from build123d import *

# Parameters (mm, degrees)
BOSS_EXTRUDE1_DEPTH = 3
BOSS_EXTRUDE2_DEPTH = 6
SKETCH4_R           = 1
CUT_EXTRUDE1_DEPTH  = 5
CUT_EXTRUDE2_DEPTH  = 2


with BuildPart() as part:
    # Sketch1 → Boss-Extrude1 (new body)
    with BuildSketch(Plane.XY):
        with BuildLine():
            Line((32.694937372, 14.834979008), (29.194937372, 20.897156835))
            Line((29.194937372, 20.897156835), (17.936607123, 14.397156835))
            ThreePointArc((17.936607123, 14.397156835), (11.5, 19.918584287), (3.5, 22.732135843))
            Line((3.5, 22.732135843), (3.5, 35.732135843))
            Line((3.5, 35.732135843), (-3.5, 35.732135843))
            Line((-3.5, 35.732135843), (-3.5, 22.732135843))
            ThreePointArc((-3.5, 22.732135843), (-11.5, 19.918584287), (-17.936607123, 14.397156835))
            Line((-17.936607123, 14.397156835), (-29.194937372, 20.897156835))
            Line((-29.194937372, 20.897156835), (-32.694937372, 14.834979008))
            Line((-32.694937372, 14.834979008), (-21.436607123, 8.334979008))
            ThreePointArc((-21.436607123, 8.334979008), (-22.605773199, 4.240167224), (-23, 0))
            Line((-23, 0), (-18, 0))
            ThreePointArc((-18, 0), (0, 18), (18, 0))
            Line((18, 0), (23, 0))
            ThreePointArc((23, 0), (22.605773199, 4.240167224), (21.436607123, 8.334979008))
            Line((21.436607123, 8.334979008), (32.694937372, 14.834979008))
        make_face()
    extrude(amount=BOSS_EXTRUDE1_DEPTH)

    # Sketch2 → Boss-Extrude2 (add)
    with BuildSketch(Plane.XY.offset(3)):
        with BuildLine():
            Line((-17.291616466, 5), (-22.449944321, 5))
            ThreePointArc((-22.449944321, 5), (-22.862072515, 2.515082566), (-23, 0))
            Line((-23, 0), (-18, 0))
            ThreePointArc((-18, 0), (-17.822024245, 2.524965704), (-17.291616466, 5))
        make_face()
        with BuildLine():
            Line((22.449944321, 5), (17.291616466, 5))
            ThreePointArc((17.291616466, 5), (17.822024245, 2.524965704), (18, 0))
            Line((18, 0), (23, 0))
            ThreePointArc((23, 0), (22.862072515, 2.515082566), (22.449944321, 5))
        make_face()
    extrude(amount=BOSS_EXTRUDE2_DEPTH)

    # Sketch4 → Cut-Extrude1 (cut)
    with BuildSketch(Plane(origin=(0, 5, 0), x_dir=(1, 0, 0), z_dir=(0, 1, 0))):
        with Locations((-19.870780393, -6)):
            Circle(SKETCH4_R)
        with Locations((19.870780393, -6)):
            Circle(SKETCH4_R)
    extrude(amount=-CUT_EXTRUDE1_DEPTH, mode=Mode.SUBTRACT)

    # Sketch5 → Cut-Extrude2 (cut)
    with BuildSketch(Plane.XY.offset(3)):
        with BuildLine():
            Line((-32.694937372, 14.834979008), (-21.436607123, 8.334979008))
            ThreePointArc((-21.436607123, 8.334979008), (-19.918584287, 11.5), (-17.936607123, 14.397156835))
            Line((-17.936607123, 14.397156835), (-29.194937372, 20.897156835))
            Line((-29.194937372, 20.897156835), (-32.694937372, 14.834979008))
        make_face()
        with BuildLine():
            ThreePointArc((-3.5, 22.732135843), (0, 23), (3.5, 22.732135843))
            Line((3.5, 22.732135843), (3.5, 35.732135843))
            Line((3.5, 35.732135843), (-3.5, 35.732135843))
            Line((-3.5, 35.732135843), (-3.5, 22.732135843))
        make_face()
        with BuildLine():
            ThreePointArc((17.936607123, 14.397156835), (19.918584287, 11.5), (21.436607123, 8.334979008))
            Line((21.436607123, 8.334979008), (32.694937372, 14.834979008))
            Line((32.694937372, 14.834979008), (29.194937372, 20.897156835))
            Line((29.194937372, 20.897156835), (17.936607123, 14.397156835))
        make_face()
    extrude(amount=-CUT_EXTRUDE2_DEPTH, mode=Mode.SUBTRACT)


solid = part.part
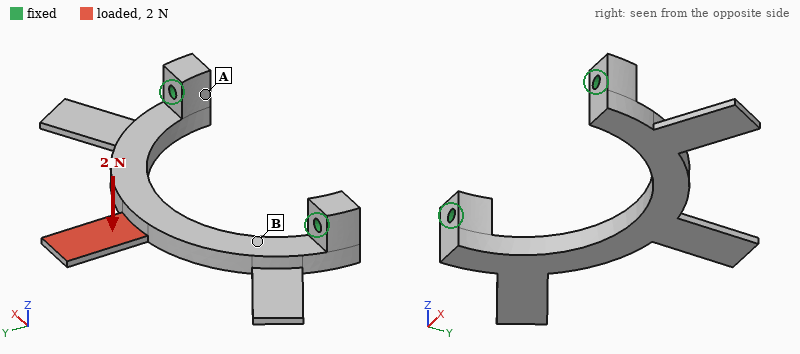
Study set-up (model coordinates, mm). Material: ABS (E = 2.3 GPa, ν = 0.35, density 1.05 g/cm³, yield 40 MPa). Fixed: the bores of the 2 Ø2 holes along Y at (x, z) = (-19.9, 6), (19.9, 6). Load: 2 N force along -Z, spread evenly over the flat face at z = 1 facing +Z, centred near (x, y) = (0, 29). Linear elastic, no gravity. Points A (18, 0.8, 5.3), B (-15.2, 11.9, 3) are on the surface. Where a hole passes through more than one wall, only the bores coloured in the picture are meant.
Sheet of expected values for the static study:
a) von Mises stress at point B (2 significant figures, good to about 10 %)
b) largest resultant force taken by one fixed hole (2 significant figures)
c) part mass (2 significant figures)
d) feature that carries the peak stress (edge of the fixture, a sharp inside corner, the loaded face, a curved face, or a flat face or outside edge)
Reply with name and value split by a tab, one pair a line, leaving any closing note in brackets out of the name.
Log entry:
von Mises stress at point B	2.3 MPa
largest resultant force taken by one fixed hole	1.0 N
part mass	1.6 g
feature that carries the peak stress	a flat face or outside edge
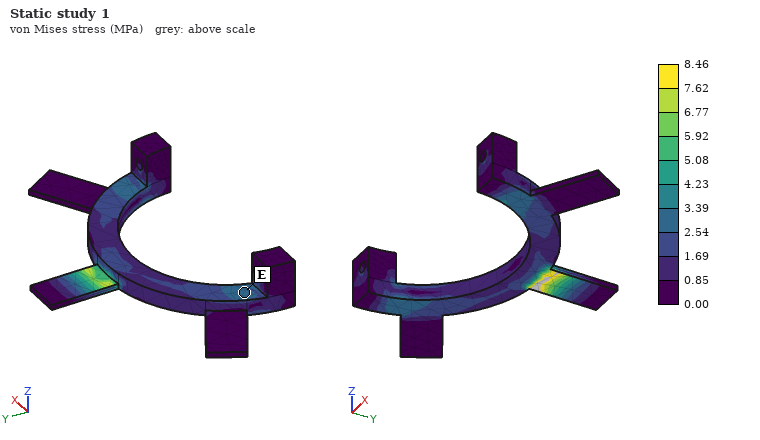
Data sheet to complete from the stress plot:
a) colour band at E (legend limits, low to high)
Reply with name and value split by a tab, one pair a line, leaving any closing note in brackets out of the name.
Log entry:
colour band at E	2.54 to 3.39 MPa
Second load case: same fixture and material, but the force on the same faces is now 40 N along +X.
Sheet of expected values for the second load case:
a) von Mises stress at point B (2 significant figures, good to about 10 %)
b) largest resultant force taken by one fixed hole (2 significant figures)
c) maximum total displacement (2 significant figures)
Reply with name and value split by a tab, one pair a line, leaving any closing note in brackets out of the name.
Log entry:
von Mises stress at point B	4.0 MPa
largest resultant force taken by one fixed hole	31 N
maximum total displacement	0.54 mm
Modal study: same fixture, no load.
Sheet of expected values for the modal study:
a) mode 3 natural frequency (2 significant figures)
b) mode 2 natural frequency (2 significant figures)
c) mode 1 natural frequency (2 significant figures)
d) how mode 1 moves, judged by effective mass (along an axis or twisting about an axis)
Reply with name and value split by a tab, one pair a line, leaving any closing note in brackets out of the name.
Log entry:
mode 3 natural frequency	1300 Hz
mode 2 natural frequency	1300 Hz
mode 1 natural frequency	780 Hz
how mode 1 moves, judged by effective mass	along Z
